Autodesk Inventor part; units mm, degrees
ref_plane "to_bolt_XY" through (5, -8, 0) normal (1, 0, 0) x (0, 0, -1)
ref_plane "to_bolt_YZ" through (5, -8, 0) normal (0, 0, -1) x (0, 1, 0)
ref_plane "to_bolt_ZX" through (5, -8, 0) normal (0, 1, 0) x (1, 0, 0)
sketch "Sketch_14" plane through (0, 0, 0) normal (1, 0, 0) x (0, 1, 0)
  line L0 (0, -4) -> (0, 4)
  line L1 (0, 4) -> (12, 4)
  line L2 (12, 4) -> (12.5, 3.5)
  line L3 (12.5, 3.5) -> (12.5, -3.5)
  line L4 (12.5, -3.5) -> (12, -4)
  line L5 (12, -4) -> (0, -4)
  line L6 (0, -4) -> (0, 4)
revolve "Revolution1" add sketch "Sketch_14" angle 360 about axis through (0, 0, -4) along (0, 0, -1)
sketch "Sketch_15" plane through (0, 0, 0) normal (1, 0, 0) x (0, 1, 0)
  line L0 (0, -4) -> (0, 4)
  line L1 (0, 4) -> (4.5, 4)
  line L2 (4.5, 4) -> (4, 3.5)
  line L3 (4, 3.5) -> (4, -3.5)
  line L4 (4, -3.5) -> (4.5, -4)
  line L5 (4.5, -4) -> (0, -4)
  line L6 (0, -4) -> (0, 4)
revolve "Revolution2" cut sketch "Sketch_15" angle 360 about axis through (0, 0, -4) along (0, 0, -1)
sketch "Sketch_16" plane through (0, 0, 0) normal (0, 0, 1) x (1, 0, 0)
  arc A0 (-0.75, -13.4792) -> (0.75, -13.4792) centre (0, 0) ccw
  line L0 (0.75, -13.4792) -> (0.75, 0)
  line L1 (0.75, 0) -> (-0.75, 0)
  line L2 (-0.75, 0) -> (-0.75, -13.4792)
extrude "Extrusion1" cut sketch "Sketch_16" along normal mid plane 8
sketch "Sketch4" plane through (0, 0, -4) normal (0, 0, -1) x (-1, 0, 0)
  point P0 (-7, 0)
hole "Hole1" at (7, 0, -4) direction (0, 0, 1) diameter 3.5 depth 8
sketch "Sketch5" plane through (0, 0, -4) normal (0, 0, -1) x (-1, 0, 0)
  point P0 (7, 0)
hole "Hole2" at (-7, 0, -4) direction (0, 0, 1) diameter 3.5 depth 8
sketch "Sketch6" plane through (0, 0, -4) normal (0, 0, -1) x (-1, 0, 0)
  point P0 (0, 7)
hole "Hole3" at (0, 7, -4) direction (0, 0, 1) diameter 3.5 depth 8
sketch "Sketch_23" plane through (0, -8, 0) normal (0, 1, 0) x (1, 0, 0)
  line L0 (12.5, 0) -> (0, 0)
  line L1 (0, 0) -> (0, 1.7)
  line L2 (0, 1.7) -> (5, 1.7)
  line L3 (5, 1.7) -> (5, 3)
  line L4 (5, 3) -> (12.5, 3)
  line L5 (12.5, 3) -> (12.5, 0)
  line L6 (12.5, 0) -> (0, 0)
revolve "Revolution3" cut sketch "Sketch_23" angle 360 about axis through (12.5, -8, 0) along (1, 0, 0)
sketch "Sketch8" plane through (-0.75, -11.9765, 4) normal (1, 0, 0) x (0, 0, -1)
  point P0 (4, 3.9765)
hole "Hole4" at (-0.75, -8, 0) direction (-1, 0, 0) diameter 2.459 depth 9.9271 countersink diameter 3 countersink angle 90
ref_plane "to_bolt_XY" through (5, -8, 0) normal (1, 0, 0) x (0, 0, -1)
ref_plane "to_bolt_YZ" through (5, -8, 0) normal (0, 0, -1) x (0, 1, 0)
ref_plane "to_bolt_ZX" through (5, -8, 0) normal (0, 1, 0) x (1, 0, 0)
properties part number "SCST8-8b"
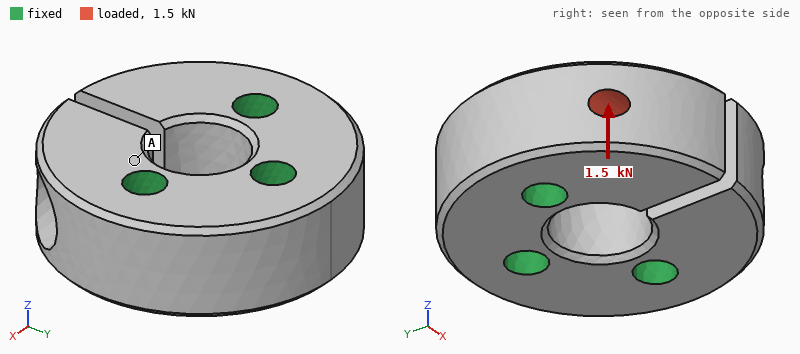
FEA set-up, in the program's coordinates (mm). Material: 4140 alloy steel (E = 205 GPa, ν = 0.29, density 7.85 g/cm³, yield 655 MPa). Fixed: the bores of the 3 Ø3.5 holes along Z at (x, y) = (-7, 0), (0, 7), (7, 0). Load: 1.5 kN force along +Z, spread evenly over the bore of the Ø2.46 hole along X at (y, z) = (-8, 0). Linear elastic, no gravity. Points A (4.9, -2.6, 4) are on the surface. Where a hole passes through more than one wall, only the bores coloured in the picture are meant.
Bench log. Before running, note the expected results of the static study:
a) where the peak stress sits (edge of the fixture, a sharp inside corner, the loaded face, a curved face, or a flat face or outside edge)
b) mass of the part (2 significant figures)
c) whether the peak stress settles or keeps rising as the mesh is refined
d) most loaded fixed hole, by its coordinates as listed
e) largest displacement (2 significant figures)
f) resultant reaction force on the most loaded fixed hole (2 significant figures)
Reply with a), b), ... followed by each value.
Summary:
a) edge of the fixture
b) 23 g
c) keeps rising
d) (-7, 0)
e) 9.6 µm
f) 1.5 kN
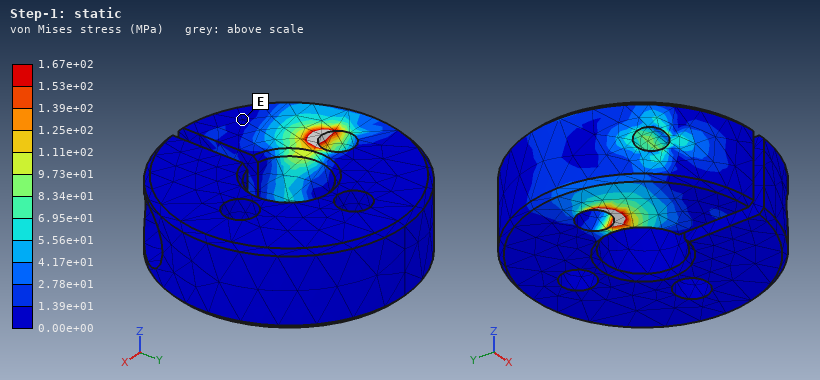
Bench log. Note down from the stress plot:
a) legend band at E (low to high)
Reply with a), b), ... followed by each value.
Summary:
a) 0.00e+00 to 1.39e+01 MPa
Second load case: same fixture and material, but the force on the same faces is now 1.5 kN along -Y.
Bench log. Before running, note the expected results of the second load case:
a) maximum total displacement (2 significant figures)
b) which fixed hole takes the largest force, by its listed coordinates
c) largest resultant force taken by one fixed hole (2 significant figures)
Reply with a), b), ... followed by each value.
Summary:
a) 4.0 µm
b) (-7, 0)
c) 1.5 kN
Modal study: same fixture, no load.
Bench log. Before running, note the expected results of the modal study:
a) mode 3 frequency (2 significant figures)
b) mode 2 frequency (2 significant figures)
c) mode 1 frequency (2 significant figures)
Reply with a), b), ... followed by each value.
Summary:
a) 36 kHz
b) 35 kHz
c) 35 kHz
